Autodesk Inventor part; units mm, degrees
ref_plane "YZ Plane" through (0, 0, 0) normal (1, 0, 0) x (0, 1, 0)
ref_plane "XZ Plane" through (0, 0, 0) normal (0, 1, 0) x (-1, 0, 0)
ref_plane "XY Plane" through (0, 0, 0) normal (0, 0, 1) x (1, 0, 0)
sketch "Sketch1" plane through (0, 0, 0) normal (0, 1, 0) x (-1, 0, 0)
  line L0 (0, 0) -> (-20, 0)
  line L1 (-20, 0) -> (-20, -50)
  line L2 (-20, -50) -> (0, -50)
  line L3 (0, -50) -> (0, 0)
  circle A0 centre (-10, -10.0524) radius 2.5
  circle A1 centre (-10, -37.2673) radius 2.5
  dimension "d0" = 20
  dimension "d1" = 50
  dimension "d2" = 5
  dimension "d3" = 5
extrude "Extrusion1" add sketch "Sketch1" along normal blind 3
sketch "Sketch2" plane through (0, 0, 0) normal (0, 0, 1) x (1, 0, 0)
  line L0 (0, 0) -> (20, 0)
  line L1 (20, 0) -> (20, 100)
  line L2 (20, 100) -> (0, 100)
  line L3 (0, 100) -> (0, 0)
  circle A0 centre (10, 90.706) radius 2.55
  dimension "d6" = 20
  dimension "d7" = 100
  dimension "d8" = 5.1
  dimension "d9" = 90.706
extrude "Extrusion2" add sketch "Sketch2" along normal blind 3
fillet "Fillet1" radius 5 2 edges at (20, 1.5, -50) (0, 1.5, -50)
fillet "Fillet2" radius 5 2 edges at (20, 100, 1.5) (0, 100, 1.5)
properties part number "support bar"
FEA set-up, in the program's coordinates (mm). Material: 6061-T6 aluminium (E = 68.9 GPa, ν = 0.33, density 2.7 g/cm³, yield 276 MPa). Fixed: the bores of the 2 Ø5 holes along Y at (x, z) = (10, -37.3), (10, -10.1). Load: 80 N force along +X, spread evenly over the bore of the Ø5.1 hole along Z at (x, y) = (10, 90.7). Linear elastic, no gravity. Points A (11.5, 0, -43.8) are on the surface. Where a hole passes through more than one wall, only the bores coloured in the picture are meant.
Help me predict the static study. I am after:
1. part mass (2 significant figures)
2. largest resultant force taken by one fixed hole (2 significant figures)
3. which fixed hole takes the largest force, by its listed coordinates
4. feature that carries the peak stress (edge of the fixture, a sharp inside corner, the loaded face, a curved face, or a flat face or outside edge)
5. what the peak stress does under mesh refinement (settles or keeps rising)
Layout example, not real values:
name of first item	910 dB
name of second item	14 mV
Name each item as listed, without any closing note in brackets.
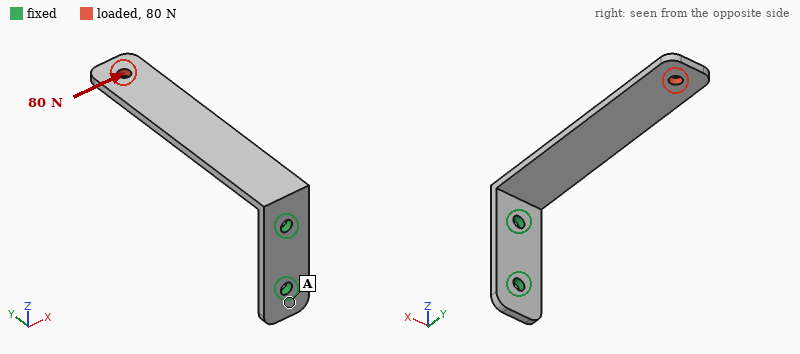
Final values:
part mass	24 g
largest resultant force taken by one fixed hole	100 N
which fixed hole takes the largest force, by its listed coordinates	(10, -10.1)
feature that carries the peak stress	edge of the fixture
what the peak stress does under mesh refinement	keeps rising
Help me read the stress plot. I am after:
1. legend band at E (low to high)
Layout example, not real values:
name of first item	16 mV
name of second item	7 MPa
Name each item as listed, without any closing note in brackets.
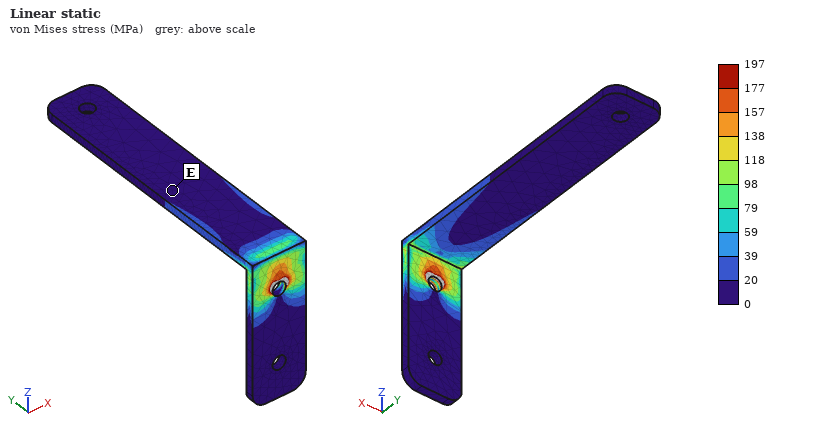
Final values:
legend band at E	0 to 20 MPa
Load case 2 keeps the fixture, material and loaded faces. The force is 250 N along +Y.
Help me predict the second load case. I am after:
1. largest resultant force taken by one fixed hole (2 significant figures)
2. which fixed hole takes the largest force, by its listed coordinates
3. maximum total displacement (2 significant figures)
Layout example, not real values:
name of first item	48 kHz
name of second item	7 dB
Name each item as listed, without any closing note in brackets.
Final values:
largest resultant force taken by one fixed hole	260 N
which fixed hole takes the largest force, by its listed coordinates	(10, -10.1)
maximum total displacement	0.44 mm
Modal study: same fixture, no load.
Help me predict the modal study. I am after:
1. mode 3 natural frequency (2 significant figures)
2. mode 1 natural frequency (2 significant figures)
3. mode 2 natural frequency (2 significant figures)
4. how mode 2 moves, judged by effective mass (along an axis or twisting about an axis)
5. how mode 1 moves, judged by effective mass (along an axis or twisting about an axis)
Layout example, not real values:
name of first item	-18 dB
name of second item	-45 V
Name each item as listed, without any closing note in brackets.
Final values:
mode 3 natural frequency	1400 Hz
mode 1 natural frequency	220 Hz
mode 2 natural frequency	520 Hz
how mode 2 moves, judged by effective mass	along X
how mode 1 moves, judged by effective mass	along Z
